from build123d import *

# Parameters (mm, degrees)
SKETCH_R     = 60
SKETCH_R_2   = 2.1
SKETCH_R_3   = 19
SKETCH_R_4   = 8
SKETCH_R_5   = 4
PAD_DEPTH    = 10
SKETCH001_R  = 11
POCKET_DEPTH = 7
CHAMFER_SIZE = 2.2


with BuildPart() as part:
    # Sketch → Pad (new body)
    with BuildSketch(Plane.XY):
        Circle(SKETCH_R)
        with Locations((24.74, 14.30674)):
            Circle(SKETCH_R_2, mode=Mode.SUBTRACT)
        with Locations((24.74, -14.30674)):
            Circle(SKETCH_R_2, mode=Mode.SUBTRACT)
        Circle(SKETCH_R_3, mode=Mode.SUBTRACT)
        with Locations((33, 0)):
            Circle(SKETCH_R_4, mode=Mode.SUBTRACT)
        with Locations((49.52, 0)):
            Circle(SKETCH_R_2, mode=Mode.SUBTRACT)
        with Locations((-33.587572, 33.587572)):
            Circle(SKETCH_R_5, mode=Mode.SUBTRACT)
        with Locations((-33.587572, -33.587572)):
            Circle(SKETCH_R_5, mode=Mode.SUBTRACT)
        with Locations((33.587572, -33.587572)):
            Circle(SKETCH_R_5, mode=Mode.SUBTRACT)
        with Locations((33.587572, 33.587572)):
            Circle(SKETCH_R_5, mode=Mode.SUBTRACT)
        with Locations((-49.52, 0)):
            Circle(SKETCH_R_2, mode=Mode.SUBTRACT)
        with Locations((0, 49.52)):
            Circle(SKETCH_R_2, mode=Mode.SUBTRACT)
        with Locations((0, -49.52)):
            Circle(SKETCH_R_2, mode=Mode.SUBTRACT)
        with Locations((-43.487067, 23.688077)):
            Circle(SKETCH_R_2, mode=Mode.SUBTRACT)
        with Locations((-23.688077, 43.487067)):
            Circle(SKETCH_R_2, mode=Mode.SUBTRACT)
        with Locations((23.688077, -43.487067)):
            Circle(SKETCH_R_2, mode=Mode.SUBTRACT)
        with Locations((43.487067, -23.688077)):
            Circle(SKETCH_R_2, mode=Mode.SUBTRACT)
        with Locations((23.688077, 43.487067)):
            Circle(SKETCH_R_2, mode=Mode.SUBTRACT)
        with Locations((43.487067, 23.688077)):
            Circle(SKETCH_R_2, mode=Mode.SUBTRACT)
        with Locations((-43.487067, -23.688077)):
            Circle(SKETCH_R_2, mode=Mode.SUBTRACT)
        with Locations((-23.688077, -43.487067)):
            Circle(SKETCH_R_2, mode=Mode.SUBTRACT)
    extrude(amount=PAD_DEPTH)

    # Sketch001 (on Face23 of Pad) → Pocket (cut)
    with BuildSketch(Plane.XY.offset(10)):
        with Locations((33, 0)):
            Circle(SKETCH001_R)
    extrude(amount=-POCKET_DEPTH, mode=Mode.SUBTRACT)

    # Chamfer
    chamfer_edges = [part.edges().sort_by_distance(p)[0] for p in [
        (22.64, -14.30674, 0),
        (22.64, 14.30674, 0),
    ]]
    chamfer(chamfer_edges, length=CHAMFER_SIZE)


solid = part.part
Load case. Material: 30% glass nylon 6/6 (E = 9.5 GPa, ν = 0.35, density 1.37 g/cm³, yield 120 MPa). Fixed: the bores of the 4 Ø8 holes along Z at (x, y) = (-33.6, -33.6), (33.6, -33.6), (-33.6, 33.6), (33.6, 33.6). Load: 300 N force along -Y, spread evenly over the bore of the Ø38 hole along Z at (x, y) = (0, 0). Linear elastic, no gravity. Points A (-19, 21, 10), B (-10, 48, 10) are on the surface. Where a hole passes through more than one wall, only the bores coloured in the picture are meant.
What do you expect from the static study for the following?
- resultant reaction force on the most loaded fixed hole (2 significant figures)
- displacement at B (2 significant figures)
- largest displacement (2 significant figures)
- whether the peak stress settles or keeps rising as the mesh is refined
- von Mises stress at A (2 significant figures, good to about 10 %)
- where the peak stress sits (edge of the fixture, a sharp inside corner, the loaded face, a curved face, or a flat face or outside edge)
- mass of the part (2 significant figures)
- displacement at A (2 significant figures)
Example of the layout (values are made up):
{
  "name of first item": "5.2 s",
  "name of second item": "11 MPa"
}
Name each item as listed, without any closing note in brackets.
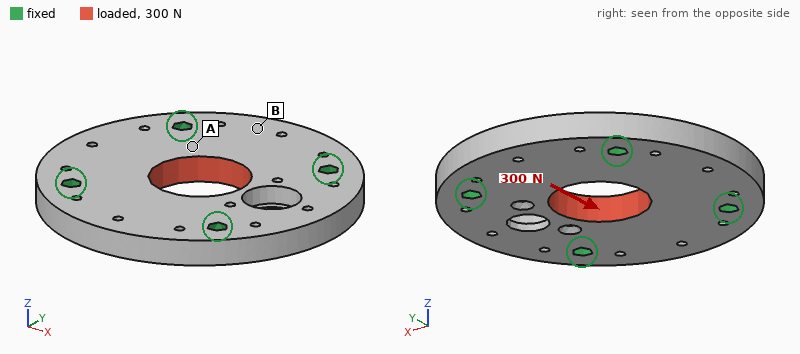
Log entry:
{
  "resultant reaction force on the most loaded fixed hole": "83 N",
  "displacement at B": "1.1 µm",
  "largest displacement": "1.7 µm",
  "whether the peak stress settles or keeps rising as the mesh is refined": "keeps rising",
  "von Mises stress at A": "0.27 MPa",
  "where the peak stress sits": "edge of the fixture",
  "mass of the part": "130 g",
  "displacement at A": "0.86 µm"
}
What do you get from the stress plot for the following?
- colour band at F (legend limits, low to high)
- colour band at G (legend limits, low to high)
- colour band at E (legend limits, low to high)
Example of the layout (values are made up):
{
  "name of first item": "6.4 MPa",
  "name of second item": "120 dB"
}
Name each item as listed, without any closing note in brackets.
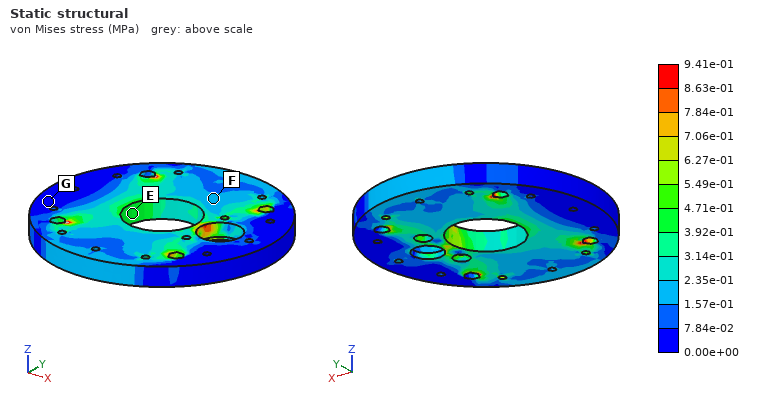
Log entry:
{
  "colour band at F": "1.57e-01 to 2.35e-01 MPa",
  "colour band at G": "0.00e+00 to 7.84e-02 MPa",
  "colour band at E": "3.92e-01 to 4.71e-01 MPa"
}
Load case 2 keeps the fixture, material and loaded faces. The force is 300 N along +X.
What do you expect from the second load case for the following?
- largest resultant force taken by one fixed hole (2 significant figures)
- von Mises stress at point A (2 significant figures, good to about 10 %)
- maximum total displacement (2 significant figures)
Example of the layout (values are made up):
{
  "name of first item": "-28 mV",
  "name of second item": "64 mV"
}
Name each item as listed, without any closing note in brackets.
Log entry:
{
  "largest resultant force taken by one fixed hole": "78 N",
  "von Mises stress at point A": "0.27 MPa",
  "maximum total displacement": "3.1 µm"
}
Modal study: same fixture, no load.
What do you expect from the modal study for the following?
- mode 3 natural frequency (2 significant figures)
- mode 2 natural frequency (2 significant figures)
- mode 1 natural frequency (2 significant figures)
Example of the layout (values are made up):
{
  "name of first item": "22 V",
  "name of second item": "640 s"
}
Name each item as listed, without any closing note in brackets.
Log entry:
{
  "mode 3 natural frequency": "4200 Hz",
  "mode 2 natural frequency": "4200 Hz",
  "mode 1 natural frequency": "4000 Hz"
}
